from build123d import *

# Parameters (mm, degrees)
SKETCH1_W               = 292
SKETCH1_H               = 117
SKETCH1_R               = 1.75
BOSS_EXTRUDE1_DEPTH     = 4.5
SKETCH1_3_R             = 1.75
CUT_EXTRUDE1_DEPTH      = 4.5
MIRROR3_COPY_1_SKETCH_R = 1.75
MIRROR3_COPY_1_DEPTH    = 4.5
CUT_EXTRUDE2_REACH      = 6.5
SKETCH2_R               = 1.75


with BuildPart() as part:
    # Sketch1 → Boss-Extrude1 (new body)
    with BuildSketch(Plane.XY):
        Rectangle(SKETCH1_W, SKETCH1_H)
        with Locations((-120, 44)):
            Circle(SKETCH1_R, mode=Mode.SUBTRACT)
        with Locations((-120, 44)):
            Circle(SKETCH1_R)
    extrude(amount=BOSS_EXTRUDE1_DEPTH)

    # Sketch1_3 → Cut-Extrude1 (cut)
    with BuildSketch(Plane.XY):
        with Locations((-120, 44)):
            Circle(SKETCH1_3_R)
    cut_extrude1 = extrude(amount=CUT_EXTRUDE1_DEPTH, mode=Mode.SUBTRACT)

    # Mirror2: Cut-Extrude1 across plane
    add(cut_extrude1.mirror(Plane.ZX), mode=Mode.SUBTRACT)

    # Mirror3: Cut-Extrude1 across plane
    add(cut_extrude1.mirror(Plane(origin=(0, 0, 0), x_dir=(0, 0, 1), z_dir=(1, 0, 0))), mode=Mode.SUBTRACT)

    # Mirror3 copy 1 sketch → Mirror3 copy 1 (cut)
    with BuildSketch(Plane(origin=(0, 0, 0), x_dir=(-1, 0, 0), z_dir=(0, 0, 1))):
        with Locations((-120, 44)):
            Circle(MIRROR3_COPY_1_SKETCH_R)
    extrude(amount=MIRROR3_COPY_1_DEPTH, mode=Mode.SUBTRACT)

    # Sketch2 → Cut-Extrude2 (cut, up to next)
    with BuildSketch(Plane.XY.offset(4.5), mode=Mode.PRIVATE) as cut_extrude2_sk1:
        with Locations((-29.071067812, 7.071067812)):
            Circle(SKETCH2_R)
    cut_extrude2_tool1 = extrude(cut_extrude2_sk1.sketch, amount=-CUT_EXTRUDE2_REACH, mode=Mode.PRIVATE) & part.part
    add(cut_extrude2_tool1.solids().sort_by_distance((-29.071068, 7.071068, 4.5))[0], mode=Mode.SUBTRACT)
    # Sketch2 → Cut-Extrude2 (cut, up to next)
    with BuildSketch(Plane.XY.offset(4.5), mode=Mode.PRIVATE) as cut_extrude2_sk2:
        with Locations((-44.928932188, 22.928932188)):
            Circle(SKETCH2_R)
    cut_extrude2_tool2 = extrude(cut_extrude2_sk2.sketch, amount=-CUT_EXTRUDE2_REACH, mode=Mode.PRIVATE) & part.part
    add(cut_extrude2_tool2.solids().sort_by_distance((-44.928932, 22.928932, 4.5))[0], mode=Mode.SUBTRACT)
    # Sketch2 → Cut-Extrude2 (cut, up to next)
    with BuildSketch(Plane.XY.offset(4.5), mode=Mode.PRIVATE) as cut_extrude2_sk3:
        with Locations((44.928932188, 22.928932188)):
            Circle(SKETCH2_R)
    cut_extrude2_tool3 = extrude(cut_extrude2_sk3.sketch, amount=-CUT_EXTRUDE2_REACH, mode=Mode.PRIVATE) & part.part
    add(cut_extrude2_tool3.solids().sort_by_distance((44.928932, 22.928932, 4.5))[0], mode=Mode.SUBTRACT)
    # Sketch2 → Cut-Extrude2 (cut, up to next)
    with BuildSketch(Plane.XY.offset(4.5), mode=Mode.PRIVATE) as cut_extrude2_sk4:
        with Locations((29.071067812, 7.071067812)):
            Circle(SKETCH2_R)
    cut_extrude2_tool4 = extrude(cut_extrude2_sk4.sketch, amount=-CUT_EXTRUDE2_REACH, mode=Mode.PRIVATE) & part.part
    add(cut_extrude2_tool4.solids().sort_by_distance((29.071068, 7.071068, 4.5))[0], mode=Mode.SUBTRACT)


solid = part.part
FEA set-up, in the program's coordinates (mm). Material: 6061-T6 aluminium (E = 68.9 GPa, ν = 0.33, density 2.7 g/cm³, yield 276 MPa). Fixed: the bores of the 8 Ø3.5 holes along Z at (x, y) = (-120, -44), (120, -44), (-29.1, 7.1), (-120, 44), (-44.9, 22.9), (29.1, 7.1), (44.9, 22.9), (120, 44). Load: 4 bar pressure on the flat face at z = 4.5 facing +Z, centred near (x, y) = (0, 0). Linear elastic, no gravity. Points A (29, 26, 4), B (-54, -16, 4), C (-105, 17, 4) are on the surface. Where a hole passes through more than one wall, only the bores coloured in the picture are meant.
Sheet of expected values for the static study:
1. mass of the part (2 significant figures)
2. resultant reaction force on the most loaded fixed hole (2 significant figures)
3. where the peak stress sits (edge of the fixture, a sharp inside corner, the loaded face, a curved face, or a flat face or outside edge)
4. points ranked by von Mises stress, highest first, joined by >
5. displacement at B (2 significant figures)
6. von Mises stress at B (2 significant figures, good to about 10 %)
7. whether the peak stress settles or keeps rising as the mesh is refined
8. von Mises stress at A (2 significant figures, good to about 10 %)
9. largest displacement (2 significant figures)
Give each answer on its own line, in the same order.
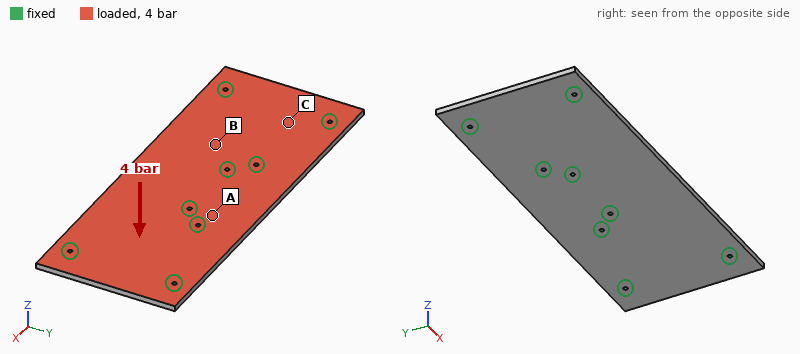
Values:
410 g
2.4 kN
edge of the fixture
B > A > C
0.38 mm
76 MPa
keeps rising
39 MPa
1.5 mm
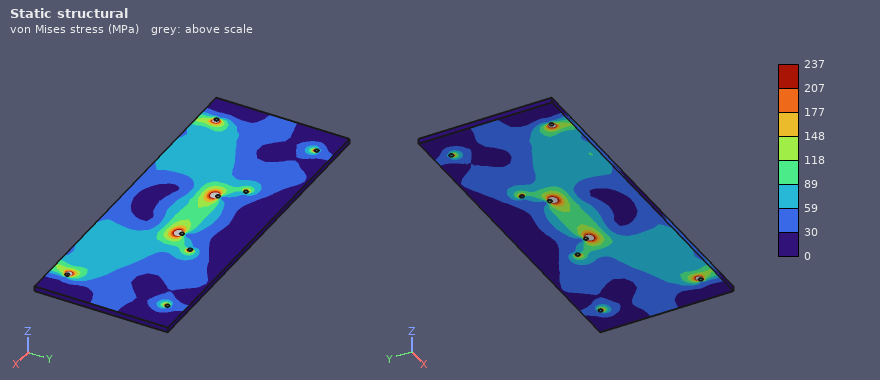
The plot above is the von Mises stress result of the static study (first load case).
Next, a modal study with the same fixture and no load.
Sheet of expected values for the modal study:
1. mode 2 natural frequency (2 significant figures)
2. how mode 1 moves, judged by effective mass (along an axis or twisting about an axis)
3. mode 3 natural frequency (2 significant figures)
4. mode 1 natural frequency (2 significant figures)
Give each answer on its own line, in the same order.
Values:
1500 Hz
along Z
2000 Hz
990 Hz
